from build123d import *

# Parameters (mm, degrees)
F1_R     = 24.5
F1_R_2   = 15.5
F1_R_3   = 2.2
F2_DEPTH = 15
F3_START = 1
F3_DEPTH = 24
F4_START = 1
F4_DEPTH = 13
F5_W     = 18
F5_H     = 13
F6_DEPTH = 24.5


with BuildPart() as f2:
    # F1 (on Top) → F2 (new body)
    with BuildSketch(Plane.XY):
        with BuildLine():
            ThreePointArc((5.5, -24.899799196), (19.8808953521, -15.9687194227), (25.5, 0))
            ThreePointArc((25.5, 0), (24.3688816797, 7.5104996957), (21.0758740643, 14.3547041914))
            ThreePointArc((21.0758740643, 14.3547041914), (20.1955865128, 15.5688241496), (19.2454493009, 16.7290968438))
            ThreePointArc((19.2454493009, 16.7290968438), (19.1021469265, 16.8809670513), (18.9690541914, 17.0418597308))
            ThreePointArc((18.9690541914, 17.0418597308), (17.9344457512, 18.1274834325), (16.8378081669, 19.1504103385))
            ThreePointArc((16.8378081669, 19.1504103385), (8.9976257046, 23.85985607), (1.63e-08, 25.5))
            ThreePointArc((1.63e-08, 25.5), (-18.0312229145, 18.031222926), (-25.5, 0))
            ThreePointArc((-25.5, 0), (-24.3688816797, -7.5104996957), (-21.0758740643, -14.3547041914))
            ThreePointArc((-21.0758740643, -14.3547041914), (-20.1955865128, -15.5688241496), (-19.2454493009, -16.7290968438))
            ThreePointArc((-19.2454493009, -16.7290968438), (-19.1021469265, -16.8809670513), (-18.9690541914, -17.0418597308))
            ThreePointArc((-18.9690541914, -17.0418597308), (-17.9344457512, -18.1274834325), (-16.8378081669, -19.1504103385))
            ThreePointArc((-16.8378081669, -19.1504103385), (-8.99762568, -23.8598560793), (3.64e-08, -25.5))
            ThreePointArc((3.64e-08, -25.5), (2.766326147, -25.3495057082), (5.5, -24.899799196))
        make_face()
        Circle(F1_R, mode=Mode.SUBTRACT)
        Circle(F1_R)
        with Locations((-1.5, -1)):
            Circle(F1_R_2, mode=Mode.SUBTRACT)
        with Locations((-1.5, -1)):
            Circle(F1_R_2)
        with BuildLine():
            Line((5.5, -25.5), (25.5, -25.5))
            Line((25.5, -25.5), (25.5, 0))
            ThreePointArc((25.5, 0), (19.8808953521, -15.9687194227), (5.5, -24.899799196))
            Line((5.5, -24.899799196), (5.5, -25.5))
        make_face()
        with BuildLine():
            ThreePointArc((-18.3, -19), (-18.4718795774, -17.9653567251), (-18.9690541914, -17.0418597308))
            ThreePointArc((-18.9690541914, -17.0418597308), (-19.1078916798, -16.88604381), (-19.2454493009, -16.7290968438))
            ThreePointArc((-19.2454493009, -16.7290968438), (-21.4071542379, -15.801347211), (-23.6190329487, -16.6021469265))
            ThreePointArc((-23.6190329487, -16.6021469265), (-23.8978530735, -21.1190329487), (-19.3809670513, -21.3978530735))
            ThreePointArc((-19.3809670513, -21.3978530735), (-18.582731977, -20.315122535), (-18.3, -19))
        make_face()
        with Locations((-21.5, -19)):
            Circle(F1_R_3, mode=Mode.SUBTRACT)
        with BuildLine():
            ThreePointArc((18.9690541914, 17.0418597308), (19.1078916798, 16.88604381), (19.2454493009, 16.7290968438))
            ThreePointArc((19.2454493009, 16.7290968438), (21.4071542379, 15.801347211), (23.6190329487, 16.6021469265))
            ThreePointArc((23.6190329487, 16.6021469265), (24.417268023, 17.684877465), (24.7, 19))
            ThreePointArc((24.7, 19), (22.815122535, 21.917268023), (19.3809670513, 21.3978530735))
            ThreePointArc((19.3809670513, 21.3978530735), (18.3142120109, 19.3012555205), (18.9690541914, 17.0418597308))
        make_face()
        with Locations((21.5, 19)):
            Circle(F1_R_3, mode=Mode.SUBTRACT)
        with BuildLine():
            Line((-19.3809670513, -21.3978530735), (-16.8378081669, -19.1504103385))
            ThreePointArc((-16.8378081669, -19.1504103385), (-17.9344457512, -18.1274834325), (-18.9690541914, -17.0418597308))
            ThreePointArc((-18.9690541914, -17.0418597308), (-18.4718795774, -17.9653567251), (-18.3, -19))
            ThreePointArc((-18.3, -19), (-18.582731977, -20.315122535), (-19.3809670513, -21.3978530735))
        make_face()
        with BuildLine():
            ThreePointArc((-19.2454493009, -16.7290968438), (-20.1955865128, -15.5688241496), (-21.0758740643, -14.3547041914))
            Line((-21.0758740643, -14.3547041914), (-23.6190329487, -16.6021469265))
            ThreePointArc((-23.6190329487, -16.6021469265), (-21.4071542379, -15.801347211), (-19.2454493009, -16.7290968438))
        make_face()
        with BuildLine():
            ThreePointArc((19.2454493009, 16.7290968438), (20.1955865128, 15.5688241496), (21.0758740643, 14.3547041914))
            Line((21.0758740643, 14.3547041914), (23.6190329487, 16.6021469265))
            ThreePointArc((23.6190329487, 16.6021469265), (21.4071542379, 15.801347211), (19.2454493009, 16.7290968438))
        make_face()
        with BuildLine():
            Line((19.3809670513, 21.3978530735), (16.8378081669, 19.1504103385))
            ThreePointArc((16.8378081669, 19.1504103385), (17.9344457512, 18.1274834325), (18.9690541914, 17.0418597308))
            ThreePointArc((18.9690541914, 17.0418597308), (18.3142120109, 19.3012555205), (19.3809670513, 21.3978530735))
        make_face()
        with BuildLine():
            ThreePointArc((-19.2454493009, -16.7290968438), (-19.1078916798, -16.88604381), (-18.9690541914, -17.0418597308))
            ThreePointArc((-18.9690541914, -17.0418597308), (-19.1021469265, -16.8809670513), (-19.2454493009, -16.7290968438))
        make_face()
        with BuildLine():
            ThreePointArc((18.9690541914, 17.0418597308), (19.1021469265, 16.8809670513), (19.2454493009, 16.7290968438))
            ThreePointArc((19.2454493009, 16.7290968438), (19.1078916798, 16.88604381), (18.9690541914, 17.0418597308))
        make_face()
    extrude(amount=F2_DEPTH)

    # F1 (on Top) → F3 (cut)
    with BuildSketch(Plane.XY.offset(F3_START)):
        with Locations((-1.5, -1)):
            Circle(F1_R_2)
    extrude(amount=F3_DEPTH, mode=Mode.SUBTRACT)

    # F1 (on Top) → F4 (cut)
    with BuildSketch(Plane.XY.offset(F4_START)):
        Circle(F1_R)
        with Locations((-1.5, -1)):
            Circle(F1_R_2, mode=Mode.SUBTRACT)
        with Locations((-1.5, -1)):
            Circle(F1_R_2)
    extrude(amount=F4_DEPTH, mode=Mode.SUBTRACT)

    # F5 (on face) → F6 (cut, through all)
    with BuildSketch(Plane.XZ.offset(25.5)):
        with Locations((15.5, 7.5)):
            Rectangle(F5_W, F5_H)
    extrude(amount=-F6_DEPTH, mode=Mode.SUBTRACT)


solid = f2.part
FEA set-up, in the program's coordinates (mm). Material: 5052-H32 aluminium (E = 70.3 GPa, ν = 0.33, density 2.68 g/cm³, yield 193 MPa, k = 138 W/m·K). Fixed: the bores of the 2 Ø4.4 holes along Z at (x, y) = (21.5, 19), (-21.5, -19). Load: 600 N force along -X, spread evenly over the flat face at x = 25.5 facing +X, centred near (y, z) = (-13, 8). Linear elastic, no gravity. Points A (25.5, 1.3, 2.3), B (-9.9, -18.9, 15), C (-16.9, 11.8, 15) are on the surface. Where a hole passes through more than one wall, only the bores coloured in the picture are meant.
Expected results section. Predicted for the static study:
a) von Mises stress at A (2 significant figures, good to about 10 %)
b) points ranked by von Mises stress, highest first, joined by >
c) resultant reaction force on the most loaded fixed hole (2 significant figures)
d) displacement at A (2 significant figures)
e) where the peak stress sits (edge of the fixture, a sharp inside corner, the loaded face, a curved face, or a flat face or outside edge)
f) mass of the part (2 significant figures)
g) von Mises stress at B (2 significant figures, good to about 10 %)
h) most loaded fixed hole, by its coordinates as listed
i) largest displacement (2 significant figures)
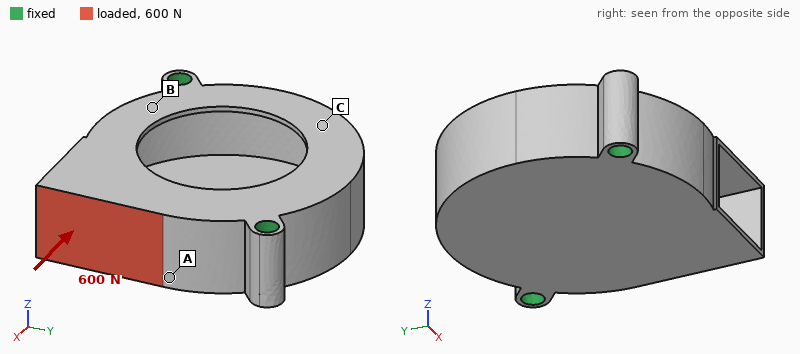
47 MPa
A > B > C
430 N
15 µm
a flat face or outside edge
17 g
31 MPa
(-21.5, -19)
87 µm
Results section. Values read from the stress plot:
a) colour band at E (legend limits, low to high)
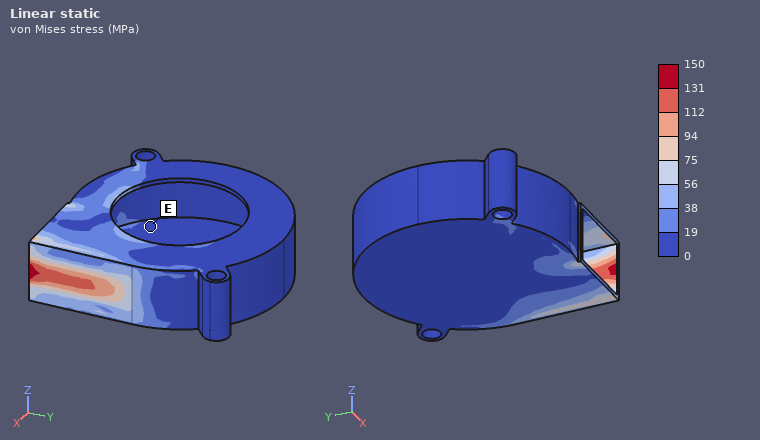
0 to 19 MPa
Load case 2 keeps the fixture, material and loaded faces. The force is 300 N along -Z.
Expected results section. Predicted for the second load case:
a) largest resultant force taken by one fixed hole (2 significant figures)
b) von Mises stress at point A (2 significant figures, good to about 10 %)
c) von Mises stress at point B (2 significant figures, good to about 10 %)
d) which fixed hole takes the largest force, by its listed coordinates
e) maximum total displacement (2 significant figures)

290 N
33 MPa
8.0 MPa
(21.5, 19)
95 µm
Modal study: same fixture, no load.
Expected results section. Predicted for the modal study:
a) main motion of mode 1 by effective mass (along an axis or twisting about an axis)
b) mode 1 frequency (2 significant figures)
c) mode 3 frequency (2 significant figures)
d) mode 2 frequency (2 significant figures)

along Z
3500 Hz
6100 Hz
5700 Hz
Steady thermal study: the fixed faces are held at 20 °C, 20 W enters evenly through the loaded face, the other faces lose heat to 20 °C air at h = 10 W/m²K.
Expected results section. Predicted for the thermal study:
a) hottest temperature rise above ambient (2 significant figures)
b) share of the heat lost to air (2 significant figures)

73 K
10 %
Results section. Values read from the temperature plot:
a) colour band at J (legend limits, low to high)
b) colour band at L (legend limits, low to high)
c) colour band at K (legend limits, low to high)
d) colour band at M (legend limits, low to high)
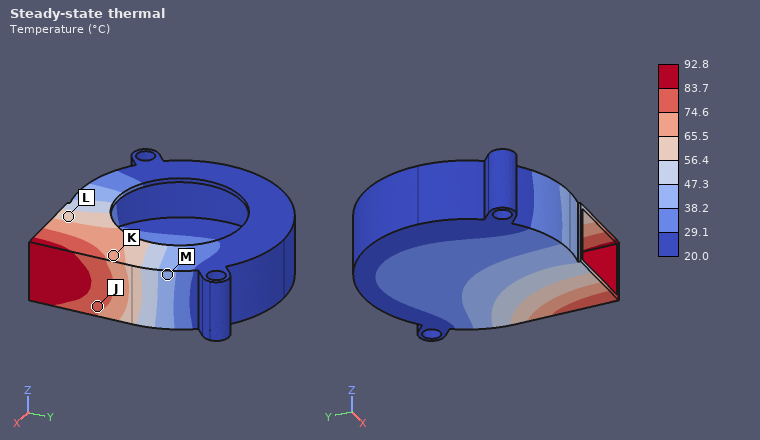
74.6 to 83.7 °C
56.4 to 65.5 °C
65.5 to 74.6 °C
38.2 to 47.3 °C
